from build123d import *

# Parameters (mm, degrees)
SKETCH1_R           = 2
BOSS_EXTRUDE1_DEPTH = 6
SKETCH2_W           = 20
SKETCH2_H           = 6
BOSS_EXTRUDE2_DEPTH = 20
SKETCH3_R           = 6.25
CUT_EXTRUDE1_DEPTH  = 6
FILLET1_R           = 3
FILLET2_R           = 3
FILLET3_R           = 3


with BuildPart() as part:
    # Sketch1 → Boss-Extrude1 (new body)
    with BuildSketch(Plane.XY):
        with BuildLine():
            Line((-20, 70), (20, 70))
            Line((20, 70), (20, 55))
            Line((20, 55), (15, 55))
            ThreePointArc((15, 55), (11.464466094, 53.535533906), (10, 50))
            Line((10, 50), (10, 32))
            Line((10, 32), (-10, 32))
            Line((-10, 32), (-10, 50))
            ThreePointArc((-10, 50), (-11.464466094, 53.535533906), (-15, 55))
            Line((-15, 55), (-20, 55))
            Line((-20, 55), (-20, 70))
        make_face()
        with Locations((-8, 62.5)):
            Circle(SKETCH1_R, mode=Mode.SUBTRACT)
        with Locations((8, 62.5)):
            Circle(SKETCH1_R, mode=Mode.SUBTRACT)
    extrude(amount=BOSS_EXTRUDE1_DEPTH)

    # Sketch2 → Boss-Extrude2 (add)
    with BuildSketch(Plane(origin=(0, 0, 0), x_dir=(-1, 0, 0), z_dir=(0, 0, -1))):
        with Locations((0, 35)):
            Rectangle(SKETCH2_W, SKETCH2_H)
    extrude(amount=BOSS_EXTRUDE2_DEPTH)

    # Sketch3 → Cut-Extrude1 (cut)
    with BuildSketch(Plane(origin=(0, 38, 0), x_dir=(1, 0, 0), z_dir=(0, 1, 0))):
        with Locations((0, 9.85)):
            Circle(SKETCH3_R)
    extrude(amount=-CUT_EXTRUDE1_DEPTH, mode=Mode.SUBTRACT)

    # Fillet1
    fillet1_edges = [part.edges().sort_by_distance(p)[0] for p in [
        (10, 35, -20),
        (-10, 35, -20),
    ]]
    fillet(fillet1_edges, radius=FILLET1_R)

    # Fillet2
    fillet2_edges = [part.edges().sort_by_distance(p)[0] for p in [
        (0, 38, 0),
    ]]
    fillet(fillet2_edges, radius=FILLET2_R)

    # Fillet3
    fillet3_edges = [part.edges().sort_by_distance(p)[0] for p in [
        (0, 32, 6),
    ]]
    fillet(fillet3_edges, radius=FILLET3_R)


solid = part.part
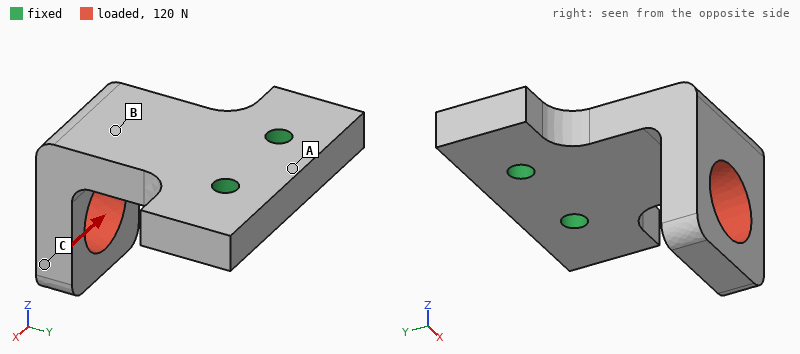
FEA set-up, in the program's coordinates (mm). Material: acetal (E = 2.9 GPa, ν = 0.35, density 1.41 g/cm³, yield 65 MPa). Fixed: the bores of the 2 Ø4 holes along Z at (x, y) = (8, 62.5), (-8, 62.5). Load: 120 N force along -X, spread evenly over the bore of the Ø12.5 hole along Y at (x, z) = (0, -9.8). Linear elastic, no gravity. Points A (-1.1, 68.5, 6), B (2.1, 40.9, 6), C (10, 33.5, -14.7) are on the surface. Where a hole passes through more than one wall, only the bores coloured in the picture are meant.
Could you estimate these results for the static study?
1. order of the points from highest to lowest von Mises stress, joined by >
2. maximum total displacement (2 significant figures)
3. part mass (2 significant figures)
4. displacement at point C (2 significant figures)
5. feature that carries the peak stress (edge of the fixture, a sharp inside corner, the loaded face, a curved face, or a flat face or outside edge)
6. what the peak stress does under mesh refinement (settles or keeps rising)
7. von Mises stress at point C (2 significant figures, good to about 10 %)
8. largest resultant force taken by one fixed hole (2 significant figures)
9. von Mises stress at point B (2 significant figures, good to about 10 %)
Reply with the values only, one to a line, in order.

B > C > A
0.62 mm
11 g
0.52 mm
edge of the fixture
keeps rising
3.2 MPa
210 N
6.9 MPa
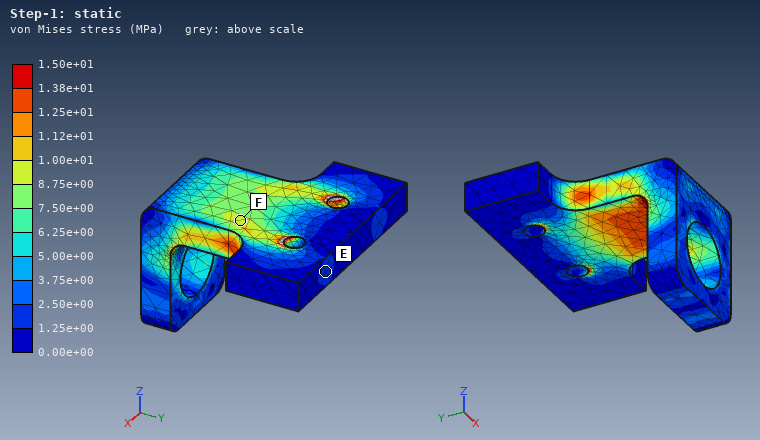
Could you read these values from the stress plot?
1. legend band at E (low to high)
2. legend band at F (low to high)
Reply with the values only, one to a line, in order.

1.25e+00 to 2.50e+00 MPa
8.75e+00 to 1.00e+01 MPa
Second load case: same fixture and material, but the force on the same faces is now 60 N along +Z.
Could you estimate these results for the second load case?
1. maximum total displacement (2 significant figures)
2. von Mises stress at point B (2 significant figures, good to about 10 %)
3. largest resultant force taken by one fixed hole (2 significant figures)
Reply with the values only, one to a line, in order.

0.57 mm
2.8 MPa
30 N
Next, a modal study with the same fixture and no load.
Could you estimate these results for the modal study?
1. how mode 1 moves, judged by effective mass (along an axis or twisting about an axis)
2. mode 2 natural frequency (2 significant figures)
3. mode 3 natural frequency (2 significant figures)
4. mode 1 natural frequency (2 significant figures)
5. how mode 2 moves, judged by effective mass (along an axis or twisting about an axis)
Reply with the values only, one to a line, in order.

along Z
1600 Hz
2400 Hz
900 Hz
along X
